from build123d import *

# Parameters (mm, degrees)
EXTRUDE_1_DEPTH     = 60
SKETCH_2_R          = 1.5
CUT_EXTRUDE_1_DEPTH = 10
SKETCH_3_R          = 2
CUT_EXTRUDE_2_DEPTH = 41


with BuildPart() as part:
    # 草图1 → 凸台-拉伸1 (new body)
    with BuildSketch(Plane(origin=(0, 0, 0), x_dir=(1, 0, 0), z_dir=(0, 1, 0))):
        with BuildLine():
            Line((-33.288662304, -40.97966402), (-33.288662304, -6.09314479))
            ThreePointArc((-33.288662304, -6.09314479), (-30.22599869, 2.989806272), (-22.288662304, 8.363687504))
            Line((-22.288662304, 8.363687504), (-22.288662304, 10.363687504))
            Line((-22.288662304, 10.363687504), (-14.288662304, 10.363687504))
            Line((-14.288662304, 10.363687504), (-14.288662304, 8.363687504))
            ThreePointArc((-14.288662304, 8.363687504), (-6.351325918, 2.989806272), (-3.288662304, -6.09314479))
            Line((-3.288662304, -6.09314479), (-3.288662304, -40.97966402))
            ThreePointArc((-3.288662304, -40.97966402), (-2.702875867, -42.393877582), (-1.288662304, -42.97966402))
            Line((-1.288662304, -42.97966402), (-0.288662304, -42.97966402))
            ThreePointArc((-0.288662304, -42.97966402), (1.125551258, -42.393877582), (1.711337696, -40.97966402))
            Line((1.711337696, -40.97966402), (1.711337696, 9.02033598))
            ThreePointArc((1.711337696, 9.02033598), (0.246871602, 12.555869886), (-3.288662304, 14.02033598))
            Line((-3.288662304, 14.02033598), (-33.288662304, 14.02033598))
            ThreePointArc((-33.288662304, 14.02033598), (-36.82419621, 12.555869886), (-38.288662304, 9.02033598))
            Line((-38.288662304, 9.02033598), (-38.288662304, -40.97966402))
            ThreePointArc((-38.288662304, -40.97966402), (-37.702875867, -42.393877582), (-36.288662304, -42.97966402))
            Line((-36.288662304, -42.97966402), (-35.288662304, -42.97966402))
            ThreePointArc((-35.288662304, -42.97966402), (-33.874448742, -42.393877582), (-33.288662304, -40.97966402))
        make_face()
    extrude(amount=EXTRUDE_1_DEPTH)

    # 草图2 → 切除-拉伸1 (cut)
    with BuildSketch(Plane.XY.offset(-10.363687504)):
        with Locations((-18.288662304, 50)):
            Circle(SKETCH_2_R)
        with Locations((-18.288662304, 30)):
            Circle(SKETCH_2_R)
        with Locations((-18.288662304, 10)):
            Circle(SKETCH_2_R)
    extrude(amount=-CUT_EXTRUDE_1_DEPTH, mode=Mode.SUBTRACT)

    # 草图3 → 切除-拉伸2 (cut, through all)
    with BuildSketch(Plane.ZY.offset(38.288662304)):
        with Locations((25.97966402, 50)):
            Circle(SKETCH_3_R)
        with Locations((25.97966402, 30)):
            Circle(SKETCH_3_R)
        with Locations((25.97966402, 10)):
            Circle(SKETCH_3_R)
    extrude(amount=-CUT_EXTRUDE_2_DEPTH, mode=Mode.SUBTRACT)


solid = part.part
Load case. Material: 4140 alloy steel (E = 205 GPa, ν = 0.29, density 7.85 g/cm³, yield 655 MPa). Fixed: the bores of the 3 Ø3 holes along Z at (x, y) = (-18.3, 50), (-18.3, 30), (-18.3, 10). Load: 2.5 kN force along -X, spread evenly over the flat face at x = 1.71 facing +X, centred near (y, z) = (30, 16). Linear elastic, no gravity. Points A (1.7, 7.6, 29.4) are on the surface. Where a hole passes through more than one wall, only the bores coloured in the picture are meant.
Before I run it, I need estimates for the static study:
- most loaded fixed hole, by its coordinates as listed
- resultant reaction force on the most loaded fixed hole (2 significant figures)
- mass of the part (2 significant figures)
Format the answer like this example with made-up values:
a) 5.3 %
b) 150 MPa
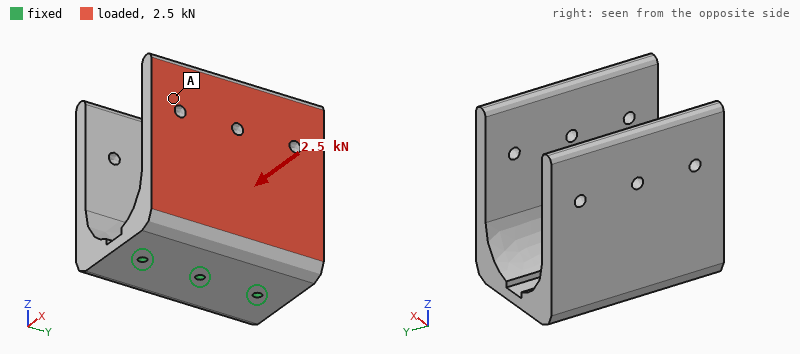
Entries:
a) (-18.3, 30)
b) 1.0 kN
c) 370 g
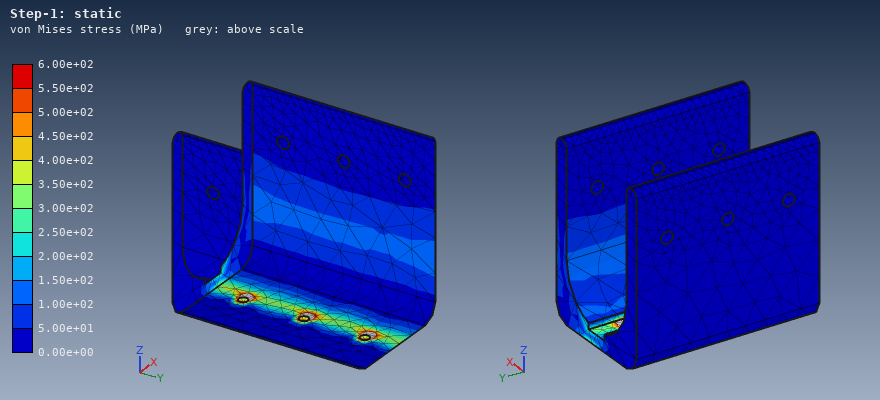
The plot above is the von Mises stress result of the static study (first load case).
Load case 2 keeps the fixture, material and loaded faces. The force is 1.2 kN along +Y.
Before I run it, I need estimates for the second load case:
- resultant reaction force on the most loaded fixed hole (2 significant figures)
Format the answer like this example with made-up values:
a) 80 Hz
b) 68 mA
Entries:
a) 1.1 kN
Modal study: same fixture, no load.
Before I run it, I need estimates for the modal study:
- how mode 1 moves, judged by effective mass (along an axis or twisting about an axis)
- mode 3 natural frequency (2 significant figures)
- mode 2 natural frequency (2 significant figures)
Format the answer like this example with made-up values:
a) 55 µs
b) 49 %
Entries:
a) along X
b) 2800 Hz
c) 1100 Hz
